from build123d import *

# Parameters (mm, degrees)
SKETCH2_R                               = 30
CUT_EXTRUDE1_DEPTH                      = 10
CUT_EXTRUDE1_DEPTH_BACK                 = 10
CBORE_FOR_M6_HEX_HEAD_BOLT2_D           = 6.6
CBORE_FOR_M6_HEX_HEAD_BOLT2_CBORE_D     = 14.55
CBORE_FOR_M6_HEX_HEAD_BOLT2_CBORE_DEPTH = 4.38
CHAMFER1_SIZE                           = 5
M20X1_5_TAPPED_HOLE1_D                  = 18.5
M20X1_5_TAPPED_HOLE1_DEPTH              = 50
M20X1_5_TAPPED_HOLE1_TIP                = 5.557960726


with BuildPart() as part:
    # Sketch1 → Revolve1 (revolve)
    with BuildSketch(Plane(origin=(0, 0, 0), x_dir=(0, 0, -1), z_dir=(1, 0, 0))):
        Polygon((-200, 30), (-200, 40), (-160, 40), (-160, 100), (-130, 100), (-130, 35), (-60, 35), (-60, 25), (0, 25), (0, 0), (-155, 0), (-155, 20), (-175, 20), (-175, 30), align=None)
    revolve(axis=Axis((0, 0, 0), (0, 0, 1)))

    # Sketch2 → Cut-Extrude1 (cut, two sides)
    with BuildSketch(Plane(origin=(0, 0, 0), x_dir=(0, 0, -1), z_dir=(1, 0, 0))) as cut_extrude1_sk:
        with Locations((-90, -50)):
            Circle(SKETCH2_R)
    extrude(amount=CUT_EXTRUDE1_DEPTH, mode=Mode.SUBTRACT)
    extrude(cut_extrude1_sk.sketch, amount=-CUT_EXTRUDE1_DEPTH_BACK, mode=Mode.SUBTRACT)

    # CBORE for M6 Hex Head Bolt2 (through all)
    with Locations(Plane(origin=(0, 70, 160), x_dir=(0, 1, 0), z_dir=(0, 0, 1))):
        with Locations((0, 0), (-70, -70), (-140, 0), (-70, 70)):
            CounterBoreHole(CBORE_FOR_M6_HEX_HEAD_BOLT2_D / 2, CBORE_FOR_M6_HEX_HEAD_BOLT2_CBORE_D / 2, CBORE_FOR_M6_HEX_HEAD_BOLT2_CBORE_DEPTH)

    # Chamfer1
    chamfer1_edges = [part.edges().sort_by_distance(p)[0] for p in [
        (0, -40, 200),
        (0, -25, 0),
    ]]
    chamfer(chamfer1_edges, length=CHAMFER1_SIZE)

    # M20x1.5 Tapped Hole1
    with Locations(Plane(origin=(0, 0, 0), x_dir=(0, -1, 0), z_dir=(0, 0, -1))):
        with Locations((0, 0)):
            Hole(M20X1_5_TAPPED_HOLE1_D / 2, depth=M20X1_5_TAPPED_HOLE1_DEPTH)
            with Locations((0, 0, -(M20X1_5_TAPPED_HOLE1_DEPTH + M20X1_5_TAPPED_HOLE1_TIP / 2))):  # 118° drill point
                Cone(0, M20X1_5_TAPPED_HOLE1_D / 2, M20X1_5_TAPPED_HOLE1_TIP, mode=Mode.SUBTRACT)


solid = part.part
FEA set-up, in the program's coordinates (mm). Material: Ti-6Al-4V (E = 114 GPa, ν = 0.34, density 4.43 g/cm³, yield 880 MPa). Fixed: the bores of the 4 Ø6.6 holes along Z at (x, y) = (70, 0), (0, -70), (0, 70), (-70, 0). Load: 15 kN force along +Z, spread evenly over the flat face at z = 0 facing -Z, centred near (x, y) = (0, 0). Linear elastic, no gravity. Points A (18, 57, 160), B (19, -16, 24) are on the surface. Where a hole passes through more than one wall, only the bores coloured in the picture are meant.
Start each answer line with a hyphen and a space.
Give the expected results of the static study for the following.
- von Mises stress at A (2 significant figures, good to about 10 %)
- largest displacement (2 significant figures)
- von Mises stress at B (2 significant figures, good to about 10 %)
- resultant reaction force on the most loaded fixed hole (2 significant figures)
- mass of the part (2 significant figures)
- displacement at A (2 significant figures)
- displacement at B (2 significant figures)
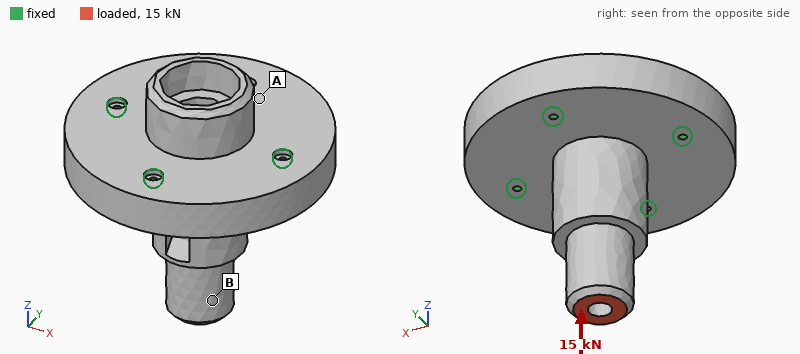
- 2.5 MPa
- 14 µm
- 8.0 MPa
- 3.8 kN
- 6.2 kg
- 2.5 µm
- 11 µm
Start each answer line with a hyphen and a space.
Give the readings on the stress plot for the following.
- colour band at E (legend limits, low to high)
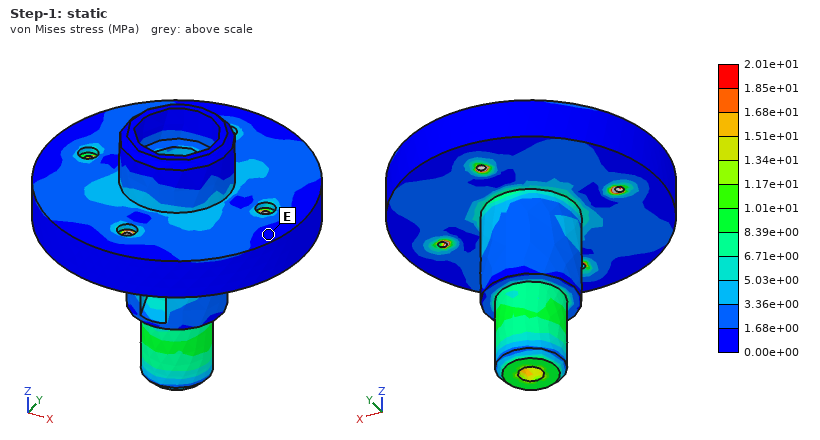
- 0.00e+00 to 1.68e+00 MPa
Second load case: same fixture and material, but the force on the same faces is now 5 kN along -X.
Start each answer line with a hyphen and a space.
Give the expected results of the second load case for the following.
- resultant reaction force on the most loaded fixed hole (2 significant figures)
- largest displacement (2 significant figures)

- 5.3 kN
- 70 µm
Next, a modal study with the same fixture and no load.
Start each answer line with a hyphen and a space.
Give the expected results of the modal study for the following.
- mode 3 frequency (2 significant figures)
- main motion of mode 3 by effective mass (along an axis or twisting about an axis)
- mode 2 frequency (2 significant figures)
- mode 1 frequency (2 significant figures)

- 4600 Hz
- along Z
- 2400 Hz
- 2400 Hz
